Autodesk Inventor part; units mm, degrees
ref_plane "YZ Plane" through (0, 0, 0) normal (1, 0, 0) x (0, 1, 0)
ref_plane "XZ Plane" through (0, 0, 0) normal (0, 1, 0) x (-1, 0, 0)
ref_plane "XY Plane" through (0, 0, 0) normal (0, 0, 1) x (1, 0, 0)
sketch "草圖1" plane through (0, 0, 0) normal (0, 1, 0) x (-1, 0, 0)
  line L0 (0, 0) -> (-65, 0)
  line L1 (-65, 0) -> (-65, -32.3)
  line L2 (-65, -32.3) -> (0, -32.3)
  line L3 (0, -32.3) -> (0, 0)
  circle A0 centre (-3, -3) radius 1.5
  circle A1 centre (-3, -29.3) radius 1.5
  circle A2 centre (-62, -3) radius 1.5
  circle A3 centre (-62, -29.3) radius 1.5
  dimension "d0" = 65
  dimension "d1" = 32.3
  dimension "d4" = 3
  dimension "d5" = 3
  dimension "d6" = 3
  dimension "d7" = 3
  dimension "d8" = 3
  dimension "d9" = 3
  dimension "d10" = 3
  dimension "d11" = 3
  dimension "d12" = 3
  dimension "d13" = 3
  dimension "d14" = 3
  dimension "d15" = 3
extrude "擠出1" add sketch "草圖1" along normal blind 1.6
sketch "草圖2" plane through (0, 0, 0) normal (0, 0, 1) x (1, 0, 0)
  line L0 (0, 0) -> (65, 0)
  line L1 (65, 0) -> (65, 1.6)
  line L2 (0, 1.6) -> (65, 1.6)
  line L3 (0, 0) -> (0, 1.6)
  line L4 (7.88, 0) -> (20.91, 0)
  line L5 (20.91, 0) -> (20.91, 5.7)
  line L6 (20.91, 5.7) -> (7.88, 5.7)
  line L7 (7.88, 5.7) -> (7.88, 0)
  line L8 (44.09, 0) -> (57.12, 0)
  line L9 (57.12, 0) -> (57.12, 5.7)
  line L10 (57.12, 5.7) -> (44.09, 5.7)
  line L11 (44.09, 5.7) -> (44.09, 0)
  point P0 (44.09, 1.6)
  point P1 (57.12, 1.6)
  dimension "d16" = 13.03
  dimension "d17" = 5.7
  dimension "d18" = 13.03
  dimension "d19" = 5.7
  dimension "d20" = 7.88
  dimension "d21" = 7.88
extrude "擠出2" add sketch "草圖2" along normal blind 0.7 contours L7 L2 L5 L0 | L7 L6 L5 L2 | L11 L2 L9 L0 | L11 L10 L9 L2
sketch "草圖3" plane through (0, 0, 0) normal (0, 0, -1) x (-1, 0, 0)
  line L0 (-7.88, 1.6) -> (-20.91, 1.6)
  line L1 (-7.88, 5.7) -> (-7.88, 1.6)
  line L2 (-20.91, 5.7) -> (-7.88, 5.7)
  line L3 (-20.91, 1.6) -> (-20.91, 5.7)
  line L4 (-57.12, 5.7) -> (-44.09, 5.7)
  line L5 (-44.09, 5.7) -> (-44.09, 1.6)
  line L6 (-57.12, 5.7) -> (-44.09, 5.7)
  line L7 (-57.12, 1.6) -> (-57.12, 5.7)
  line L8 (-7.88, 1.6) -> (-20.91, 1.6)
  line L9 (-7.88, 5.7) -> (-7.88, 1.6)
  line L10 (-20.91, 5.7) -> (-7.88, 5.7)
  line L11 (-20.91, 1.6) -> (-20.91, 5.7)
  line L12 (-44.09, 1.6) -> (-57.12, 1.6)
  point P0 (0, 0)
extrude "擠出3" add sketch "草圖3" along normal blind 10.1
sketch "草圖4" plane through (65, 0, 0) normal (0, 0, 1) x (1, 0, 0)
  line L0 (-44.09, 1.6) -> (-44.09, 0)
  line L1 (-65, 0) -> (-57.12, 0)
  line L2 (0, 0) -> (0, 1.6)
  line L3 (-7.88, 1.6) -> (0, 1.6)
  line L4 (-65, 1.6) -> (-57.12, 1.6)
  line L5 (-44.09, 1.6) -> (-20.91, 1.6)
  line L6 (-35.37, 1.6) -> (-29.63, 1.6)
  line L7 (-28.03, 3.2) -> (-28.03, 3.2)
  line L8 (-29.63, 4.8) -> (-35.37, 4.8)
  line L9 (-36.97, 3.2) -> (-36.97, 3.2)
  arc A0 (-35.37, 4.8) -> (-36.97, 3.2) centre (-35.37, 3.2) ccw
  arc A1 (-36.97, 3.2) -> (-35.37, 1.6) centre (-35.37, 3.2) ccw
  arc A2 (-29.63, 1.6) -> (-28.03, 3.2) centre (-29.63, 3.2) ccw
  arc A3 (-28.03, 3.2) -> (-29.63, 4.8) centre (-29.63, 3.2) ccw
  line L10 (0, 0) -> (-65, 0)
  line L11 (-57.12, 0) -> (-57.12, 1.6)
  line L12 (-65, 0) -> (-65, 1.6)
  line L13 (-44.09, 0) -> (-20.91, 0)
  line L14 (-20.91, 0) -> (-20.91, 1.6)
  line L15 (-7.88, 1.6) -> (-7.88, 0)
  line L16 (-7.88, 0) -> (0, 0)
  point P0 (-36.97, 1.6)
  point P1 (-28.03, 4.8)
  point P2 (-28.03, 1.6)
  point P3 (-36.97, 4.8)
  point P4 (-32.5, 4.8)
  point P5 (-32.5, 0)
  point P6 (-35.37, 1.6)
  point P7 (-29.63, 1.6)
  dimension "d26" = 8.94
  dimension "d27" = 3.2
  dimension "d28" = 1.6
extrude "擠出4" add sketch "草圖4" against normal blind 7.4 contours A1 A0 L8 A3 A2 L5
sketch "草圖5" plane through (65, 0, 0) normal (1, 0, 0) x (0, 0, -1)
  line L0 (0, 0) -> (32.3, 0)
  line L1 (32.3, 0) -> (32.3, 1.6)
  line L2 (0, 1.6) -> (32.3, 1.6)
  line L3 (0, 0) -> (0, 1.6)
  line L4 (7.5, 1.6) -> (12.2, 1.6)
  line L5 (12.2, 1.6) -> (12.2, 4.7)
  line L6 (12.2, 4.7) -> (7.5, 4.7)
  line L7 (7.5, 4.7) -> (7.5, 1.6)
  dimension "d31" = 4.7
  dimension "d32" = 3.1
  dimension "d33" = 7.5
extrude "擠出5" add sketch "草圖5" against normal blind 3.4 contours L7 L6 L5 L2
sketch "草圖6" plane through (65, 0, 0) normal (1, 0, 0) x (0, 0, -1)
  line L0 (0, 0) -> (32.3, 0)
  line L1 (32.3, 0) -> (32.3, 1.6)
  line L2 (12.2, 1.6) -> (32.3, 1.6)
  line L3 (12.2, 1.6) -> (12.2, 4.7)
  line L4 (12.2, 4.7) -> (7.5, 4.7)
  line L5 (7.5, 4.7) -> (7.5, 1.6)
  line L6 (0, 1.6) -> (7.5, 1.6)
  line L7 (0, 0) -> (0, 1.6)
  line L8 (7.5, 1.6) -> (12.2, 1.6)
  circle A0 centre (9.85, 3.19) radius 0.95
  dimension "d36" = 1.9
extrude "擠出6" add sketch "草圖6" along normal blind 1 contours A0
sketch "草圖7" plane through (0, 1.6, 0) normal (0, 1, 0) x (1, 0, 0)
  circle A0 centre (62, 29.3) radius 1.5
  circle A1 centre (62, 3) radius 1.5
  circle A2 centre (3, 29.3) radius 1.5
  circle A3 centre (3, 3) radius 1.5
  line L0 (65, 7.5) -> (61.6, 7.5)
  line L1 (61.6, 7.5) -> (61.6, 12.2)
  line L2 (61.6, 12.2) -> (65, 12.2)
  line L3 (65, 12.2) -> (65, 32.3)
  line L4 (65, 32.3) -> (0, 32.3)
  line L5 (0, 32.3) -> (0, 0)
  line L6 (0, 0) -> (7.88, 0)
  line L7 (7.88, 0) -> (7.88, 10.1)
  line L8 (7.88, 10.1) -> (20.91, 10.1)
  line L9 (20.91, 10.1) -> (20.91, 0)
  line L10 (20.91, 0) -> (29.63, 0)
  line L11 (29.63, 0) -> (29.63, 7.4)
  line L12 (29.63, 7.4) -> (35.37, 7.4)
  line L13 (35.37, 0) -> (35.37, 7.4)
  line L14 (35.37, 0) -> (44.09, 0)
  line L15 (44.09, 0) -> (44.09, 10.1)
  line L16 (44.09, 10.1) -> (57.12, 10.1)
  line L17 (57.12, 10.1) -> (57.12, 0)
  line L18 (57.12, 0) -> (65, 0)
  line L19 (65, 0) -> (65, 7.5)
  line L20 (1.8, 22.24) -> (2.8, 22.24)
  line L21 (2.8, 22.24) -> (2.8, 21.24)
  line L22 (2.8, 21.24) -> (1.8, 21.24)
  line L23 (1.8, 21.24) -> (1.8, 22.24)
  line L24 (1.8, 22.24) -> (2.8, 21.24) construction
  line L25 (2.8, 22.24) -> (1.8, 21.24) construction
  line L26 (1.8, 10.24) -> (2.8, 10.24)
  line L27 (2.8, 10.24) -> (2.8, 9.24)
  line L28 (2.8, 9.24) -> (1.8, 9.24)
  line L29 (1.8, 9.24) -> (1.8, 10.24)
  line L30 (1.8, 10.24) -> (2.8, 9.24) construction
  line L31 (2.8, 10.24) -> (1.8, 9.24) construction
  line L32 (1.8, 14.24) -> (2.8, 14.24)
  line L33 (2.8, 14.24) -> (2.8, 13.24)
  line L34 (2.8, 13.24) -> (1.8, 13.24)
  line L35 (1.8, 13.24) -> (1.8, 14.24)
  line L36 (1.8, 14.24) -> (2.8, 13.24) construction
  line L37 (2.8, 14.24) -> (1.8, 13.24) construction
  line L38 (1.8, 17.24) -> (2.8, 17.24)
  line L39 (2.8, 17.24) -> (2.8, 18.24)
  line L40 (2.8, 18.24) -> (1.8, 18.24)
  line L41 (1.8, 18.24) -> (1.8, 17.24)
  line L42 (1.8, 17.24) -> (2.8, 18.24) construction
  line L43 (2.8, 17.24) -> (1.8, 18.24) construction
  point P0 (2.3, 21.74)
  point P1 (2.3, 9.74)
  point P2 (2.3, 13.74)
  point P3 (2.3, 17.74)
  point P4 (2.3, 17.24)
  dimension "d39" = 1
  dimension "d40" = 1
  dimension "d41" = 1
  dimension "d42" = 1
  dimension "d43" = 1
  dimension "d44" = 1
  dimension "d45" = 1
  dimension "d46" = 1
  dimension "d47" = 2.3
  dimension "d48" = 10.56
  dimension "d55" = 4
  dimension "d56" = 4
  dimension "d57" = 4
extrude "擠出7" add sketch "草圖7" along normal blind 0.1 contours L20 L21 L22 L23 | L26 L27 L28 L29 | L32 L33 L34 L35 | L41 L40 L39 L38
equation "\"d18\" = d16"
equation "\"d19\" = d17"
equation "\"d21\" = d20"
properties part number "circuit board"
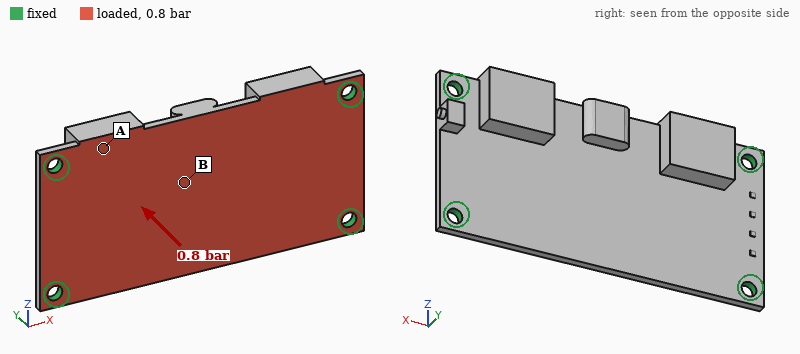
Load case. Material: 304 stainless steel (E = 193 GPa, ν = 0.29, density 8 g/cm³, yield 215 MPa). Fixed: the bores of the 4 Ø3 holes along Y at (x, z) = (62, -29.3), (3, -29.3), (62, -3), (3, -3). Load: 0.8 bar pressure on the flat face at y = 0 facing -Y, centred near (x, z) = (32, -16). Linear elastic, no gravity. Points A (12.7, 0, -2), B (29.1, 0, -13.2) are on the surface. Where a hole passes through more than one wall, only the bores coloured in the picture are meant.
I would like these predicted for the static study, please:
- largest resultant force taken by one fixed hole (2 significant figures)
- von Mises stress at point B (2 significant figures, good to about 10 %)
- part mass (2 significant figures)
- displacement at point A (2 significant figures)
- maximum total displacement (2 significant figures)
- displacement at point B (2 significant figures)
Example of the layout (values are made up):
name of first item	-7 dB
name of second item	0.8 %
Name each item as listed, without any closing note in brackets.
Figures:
largest resultant force taken by one fixed hole	42 N
von Mises stress at point B	22 MPa
part mass	38 g
displacement at point A	11 µm
maximum total displacement	43 µm
displacement at point B	38 µm
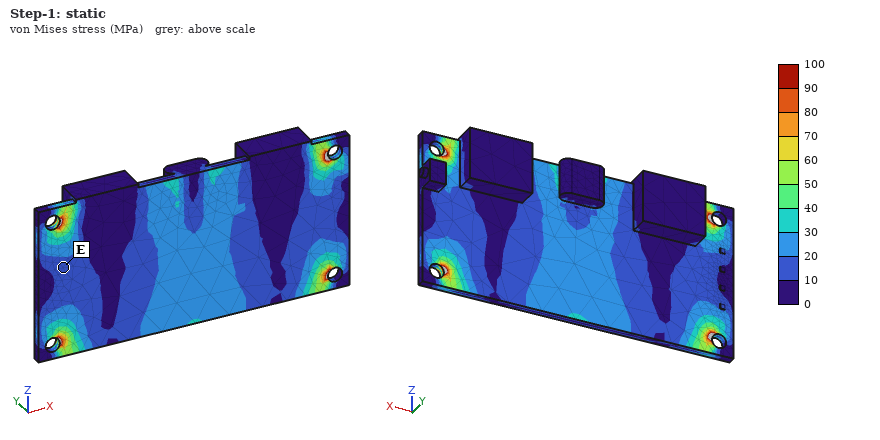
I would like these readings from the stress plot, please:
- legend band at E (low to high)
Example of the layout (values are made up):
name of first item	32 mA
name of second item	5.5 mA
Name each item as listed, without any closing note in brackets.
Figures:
legend band at E	10 to 20 MPa
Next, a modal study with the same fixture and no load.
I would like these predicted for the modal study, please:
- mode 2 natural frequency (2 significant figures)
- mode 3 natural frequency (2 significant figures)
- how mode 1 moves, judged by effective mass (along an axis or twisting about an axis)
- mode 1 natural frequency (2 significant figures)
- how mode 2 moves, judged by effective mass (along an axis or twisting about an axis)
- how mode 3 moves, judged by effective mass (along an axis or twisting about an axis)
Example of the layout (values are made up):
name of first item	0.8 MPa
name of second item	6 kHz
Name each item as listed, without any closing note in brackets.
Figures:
mode 2 natural frequency	4000 Hz
mode 3 natural frequency	5600 Hz
how mode 1 moves, judged by effective mass	along Y
mode 1 natural frequency	2000 Hz
how mode 2 moves, judged by effective mass	twisting about X
how mode 3 moves, judged by effective mass	twisting about Z
